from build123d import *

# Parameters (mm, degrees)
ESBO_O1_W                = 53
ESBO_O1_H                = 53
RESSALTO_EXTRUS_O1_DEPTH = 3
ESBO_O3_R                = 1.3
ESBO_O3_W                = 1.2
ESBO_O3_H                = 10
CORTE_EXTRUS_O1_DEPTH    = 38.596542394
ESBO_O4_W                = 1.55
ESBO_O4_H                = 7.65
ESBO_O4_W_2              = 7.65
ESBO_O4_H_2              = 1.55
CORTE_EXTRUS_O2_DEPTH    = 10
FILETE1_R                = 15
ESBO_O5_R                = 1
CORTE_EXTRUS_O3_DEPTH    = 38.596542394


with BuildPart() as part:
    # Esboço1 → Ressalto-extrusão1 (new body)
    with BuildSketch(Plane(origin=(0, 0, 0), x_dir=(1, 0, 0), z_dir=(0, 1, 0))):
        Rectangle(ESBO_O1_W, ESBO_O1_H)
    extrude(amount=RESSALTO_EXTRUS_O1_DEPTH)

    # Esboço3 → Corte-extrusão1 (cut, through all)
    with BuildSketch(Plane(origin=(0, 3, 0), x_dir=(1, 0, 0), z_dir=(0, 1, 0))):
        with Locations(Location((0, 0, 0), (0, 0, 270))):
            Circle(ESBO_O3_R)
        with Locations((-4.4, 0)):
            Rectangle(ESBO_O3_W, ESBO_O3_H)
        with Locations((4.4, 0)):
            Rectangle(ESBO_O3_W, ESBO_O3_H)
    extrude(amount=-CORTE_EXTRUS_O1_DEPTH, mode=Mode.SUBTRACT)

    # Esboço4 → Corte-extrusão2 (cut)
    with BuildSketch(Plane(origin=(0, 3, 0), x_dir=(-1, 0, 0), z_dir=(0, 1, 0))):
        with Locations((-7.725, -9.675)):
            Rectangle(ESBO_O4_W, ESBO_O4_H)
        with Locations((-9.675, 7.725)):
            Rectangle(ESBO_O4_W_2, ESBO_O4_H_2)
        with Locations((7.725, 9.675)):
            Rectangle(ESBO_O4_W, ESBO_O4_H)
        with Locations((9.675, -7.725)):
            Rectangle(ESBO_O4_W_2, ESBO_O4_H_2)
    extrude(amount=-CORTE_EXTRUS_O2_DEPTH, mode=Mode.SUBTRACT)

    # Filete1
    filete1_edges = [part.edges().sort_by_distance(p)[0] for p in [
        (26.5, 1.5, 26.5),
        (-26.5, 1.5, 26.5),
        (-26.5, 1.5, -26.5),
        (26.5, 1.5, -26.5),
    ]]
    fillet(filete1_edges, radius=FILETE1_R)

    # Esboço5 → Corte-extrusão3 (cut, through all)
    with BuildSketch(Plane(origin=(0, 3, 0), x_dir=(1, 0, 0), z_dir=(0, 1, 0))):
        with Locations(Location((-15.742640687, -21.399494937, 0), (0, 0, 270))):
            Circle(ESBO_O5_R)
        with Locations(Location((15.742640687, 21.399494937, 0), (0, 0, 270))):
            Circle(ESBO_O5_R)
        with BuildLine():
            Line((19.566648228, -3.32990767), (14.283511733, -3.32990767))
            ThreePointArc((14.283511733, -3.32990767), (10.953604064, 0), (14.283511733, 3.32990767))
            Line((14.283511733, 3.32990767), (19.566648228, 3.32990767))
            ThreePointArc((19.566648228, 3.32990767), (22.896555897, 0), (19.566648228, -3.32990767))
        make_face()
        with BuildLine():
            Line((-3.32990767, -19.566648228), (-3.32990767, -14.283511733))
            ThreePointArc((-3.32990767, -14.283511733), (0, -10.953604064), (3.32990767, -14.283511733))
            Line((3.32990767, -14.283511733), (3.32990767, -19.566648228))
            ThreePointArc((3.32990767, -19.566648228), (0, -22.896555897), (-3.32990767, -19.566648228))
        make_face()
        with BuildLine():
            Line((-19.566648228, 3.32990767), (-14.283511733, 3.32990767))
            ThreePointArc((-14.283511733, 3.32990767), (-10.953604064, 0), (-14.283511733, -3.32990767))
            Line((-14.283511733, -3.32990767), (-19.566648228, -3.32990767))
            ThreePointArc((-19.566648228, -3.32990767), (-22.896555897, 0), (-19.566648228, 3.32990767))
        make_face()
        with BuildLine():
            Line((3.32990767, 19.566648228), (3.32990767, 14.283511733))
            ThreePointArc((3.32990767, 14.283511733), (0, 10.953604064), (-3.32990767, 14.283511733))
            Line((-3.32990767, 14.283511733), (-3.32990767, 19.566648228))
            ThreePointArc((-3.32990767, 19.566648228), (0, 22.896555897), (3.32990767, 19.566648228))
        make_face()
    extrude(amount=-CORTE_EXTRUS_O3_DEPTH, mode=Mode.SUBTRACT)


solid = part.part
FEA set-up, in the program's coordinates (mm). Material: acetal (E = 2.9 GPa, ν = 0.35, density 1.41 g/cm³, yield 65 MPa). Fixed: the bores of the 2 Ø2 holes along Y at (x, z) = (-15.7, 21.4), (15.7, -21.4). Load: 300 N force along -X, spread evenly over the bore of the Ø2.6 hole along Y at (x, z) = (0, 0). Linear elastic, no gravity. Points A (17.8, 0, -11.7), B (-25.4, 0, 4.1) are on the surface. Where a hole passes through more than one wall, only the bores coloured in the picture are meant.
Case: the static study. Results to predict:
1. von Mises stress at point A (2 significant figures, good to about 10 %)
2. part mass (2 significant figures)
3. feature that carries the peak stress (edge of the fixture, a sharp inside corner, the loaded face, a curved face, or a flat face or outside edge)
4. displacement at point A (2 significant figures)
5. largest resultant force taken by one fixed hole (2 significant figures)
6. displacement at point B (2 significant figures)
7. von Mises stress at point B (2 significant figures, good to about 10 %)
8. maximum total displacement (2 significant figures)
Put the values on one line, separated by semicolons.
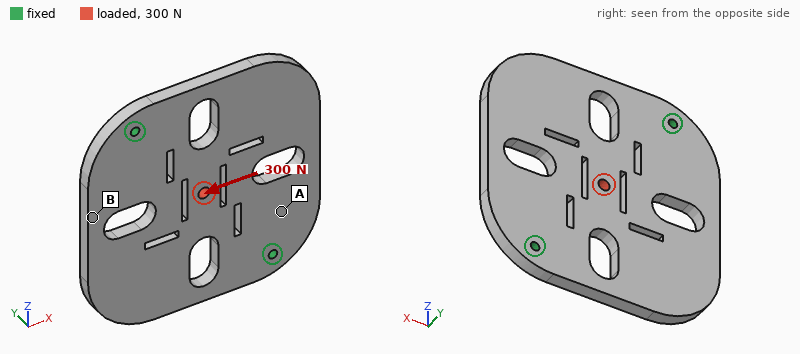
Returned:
1.8 MPa; 9.5 g; a sharp inside corner; 0.028 mm; 150 N; 0.039 mm; 3.8 MPa; 0.12 mm
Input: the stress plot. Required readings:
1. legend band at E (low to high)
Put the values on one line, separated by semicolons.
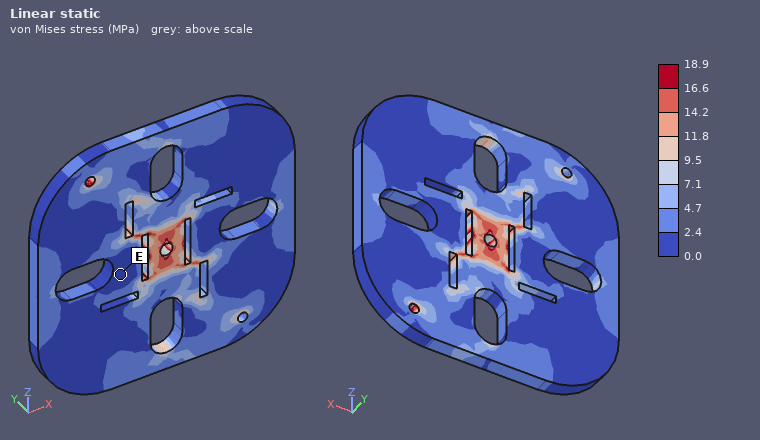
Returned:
0.0 to 2.4 MPa
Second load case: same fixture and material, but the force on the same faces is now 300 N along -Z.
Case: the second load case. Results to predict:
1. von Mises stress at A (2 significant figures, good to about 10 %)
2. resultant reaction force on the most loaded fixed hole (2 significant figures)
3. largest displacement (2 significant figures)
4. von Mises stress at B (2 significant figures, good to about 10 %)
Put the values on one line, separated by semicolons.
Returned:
1.9 MPa; 150 N; 74 µm; 3.1 MPa
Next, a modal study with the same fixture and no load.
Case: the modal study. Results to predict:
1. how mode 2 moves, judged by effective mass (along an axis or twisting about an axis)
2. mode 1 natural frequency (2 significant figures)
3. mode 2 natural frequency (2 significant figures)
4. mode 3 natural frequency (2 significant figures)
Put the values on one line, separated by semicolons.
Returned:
along Y; 530 Hz; 720 Hz; 1700 Hz
